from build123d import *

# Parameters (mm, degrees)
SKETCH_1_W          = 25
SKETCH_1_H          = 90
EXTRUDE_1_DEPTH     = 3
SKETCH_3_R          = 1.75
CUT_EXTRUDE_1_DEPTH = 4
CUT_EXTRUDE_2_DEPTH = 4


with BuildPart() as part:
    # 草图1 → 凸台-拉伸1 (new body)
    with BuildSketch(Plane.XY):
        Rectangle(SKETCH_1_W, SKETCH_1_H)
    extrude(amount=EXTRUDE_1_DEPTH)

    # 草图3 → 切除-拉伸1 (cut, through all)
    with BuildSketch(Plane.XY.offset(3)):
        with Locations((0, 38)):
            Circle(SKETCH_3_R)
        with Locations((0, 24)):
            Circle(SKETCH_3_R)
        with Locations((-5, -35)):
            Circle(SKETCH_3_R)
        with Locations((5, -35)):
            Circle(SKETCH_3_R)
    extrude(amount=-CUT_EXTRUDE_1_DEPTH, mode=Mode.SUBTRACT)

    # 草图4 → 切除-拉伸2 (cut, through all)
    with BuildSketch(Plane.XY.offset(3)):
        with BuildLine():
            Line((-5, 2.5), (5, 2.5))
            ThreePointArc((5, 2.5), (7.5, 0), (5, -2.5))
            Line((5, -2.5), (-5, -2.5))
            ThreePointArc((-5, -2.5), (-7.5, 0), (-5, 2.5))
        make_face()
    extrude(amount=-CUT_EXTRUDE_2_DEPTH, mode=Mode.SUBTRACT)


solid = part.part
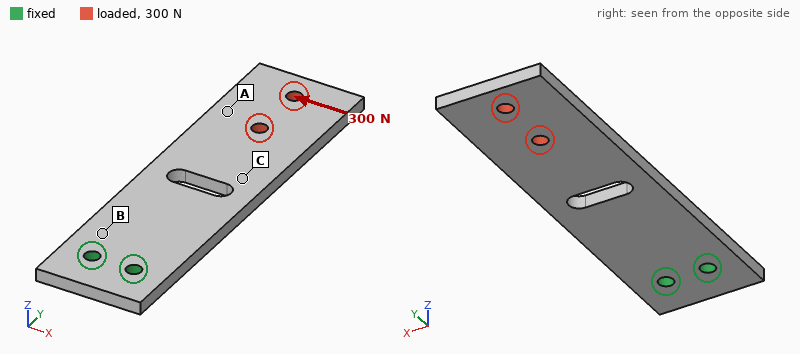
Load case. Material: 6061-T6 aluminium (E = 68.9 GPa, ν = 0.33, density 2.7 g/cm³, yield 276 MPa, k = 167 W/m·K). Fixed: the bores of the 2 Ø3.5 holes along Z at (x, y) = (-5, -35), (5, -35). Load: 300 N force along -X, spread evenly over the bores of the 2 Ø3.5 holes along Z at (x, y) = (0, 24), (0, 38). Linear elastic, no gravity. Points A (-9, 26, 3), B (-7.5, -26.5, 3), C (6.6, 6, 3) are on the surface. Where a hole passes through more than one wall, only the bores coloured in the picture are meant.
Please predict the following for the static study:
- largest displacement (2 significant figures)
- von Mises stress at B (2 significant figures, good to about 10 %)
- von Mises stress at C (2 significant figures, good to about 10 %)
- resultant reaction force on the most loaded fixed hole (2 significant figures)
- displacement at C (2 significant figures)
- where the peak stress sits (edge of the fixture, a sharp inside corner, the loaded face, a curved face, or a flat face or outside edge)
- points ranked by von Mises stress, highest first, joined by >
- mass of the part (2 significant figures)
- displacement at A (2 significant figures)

0.20 mm
38 MPa
20 MPa
1.6 kN
0.082 mm
edge of the fixture
B > C > A
17 g
0.14 mm
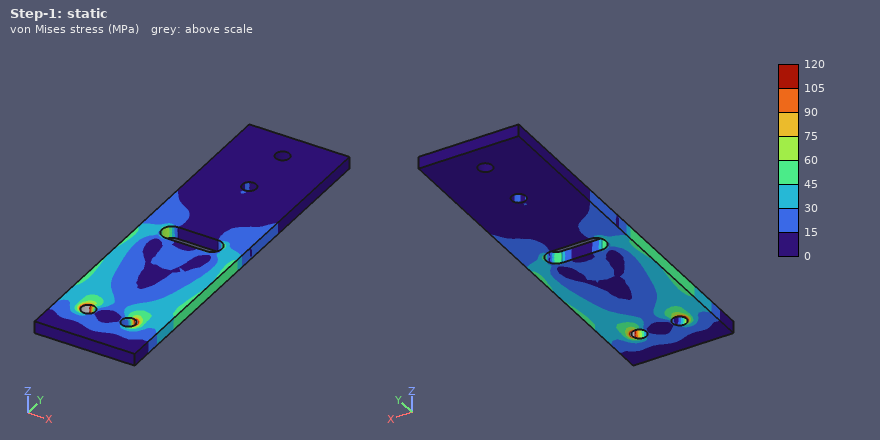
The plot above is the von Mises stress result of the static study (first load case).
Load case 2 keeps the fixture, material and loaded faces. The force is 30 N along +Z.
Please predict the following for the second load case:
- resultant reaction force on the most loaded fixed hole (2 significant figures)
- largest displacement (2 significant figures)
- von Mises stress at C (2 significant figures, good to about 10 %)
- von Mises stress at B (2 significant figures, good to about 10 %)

15 N
1.1 mm
25 MPa
44 MPa
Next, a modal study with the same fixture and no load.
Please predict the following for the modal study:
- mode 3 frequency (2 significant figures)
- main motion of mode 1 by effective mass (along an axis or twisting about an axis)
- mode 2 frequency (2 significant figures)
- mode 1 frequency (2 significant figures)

2300 Hz
along Z
2300 Hz
380 Hz
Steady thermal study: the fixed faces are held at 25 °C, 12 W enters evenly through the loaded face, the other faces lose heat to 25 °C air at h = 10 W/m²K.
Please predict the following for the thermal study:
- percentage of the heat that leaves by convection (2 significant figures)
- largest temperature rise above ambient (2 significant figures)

15 %
70 K
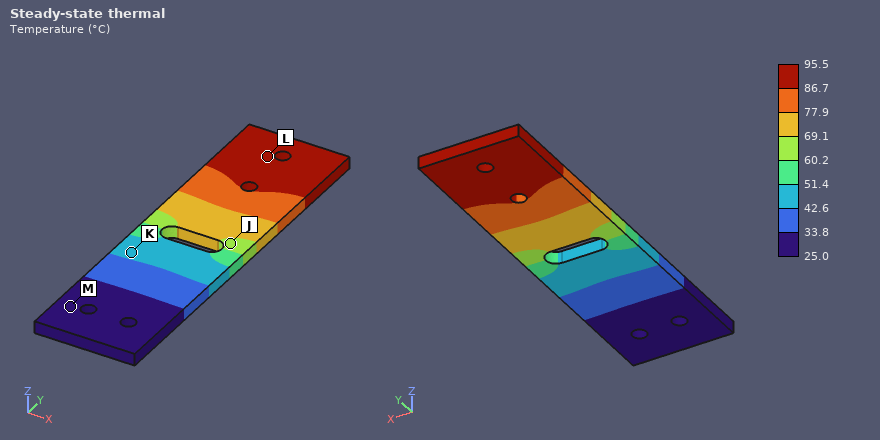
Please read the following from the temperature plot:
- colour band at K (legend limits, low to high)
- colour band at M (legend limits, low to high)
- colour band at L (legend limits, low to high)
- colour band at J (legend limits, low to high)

42.6 to 51.4 °C
25.0 to 33.8 °C
86.7 to 95.5 °C
60.2 to 69.1 °C
